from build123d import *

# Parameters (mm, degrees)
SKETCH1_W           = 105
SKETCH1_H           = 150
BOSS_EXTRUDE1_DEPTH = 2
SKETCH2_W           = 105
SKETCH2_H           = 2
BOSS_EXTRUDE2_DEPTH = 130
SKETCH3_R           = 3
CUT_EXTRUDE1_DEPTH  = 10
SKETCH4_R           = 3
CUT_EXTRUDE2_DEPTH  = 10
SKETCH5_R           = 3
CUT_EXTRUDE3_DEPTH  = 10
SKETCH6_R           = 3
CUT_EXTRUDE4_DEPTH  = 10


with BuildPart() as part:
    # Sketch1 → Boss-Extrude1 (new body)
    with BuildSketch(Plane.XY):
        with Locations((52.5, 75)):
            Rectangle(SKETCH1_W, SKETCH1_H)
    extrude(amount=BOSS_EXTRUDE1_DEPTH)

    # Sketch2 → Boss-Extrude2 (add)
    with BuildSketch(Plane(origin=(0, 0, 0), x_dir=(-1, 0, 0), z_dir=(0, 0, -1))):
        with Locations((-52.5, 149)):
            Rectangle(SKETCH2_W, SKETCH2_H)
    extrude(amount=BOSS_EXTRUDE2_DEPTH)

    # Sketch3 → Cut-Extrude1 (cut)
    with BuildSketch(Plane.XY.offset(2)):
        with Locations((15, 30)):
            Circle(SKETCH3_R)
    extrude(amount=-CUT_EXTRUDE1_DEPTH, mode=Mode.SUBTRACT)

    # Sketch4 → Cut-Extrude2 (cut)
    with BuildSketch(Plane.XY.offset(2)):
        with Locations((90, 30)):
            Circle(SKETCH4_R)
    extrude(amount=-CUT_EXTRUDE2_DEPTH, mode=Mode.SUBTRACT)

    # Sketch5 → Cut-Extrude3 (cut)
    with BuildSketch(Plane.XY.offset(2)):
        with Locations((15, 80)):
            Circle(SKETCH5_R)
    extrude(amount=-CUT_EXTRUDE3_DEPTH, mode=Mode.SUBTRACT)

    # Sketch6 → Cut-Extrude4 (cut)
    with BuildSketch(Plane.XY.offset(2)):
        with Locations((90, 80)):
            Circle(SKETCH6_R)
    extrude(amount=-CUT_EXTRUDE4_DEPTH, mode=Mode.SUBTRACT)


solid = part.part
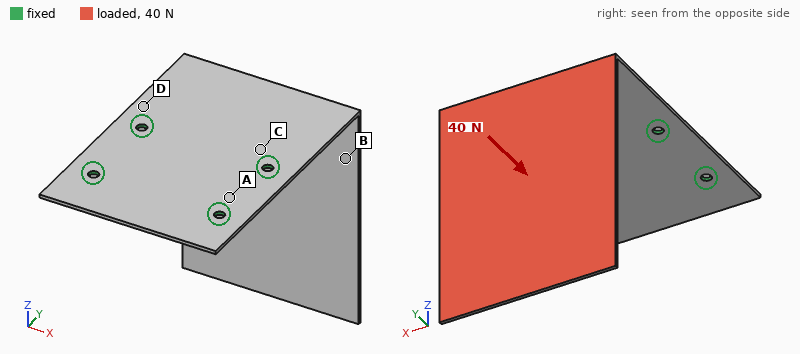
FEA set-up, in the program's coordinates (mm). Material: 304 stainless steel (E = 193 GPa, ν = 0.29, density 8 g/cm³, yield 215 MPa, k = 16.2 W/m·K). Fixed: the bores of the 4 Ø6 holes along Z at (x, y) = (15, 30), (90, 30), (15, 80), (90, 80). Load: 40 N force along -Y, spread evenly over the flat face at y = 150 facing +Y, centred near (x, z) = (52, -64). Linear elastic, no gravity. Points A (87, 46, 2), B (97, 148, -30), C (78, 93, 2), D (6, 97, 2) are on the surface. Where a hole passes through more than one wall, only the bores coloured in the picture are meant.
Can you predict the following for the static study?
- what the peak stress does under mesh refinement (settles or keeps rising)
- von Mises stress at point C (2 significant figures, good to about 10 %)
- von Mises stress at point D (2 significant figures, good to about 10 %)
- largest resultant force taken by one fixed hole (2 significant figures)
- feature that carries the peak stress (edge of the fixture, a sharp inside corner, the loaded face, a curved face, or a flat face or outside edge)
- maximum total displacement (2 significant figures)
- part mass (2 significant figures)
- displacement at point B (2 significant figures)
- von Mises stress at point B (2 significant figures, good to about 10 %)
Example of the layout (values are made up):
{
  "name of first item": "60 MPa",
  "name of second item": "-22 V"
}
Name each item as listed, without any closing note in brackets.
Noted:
{
  "what the peak stress does under mesh refinement": "keeps rising",
  "von Mises stress at point C": "34 MPa",
  "von Mises stress at point D": "41 MPa",
  "largest resultant force taken by one fixed hole": "17 N",
  "feature that carries the peak stress": "edge of the fixture",
  "maximum total displacement": "2.5 mm",
  "part mass": "470 g",
  "displacement at point B": "0.64 mm",
  "von Mises stress at point B": "21 MPa"
}
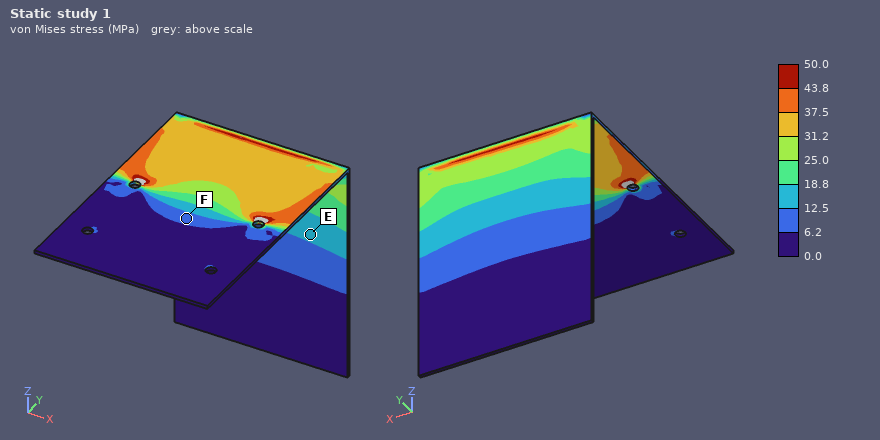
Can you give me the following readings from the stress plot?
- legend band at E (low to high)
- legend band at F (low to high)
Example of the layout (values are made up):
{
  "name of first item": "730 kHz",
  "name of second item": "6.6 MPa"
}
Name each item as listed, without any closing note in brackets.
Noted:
{
  "legend band at E": "12.5 to 18.8 MPa",
  "legend band at F": "6.2 to 12.5 MPa"
}
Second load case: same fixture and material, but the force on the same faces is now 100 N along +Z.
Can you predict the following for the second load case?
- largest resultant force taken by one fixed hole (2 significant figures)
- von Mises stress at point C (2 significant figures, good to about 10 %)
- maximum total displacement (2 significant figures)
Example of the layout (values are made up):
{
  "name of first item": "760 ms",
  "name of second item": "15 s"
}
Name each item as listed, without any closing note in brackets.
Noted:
{
  "largest resultant force taken by one fixed hole": "69 N",
  "von Mises stress at point C": "76 MPa",
  "maximum total displacement": "2.6 mm"
}
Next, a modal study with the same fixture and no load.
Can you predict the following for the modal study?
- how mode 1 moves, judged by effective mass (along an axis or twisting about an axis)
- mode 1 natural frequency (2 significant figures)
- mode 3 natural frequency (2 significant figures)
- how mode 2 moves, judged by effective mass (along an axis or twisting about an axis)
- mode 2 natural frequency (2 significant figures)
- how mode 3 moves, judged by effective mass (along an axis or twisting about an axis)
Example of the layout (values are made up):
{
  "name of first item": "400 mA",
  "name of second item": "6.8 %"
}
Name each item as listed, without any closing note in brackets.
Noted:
{
  "how mode 1 moves, judged by effective mass": "along Y",
  "mode 1 natural frequency": "50 Hz",
  "mode 3 natural frequency": "170 Hz",
  "how mode 2 moves, judged by effective mass": "along X",
  "mode 2 natural frequency": "100 Hz",
  "how mode 3 moves, judged by effective mass": "along Z"
}
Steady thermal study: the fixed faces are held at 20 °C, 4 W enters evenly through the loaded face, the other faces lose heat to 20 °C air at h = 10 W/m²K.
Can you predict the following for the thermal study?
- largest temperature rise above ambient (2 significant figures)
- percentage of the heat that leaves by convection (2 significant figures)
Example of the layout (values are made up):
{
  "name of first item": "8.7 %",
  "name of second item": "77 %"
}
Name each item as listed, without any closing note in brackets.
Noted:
{
  "largest temperature rise above ambient": "24 K",
  "percentage of the heat that leaves by convection": "94 %"
}
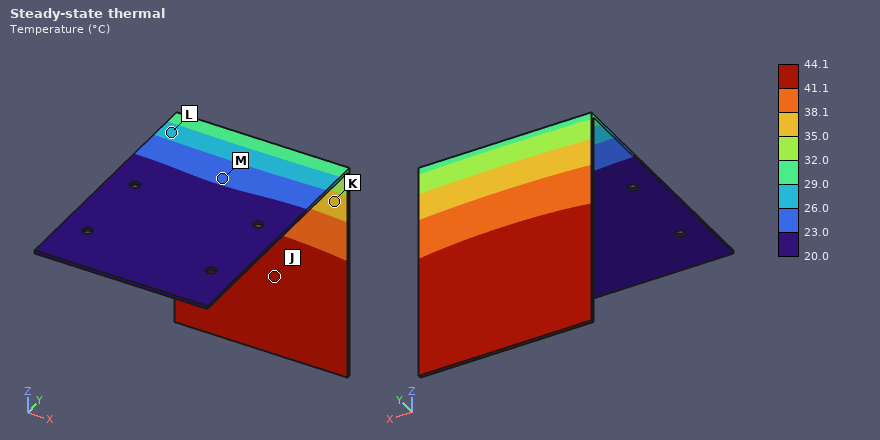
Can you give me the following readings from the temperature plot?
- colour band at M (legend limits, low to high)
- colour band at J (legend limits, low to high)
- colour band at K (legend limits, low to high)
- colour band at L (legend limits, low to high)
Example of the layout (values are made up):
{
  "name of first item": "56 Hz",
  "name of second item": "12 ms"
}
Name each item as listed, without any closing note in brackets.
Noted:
{
  "colour band at M": "23.0 to 26.0 °C",
  "colour band at J": "41.1 to 44.1 °C",
  "colour band at K": "35.0 to 38.1 °C",
  "colour band at L": "26.0 to 29.0 °C"
}
